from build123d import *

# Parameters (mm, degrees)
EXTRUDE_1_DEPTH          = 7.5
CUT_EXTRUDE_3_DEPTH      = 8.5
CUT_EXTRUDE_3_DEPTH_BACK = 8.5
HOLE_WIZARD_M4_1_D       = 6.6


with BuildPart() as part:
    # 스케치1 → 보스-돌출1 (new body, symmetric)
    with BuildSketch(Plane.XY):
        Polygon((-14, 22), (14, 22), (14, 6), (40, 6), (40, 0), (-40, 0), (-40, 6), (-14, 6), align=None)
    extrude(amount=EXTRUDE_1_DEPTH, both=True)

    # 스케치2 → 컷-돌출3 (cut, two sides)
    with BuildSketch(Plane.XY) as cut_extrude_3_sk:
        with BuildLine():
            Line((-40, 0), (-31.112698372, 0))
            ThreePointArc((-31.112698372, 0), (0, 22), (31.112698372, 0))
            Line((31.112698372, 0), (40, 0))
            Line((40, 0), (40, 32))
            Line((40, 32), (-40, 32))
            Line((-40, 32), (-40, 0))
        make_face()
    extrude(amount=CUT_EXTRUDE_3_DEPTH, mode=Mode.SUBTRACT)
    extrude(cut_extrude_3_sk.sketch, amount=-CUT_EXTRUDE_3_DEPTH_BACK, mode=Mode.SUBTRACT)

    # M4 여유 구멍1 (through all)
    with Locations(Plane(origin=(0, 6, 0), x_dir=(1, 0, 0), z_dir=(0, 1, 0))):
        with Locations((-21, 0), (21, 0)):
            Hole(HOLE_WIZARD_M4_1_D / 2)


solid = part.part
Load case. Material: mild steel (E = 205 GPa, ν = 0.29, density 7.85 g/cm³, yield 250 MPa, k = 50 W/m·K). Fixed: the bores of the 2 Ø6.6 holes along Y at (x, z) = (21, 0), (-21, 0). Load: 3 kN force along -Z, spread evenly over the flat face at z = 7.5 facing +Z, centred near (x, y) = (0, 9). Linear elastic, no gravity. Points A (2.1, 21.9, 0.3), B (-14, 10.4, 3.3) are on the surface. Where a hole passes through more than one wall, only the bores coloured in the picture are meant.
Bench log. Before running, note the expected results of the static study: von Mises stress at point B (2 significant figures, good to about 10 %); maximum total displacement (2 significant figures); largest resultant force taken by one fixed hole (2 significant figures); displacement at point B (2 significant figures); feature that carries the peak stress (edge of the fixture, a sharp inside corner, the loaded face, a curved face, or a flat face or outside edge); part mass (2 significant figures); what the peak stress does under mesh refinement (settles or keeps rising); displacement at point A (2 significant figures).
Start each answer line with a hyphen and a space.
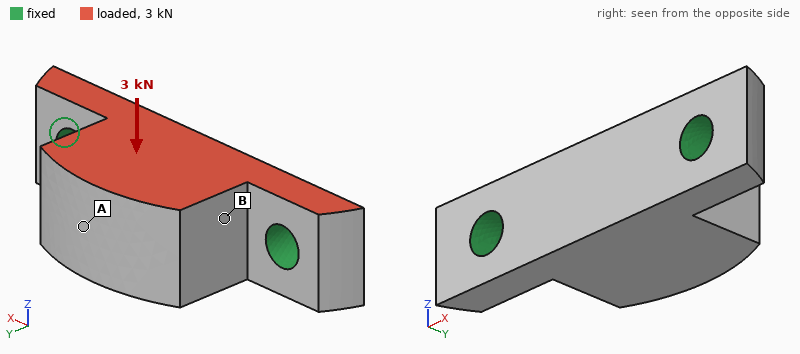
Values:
- 22 MPa
- 18 µm
- 1.5 kN
- 7.9 µm
- edge of the fixture
- 88 g
- keeps rising
- 17 µm
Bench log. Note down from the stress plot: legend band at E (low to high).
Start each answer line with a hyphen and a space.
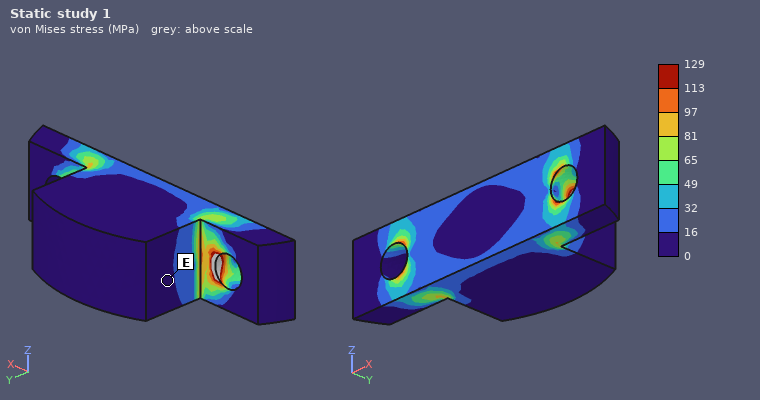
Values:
- 0 to 16 MPa
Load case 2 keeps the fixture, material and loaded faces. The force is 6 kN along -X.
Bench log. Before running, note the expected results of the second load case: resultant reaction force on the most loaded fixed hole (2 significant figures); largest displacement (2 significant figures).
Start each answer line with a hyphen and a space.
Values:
- 3.3 kN
- 6.7 µm
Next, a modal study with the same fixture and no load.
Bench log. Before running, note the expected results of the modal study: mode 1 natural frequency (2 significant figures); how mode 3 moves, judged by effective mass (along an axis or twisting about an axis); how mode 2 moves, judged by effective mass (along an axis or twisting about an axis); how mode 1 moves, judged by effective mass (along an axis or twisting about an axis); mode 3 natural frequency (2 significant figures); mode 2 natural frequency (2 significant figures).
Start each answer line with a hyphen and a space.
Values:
- 8100 Hz
- along X
- along Y
- along Z
- 22 kHz
- 18 kHz
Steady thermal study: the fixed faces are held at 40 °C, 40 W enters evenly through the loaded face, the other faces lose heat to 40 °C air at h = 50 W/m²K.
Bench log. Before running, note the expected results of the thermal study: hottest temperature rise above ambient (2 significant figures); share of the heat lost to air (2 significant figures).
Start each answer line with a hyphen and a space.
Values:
- 42 K
- 7.8 %
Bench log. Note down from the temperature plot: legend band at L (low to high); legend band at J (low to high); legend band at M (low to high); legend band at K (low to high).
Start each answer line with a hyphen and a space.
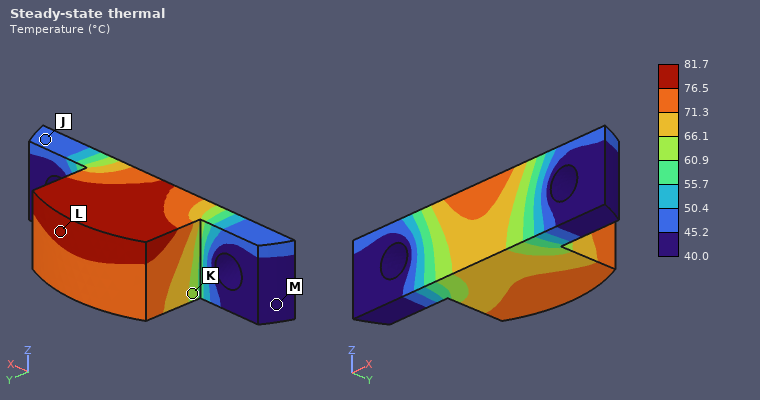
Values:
- 76.5 to 81.7 °C
- 45.2 to 50.4 °C
- 40.0 to 45.2 °C
- 60.9 to 66.1 °C
